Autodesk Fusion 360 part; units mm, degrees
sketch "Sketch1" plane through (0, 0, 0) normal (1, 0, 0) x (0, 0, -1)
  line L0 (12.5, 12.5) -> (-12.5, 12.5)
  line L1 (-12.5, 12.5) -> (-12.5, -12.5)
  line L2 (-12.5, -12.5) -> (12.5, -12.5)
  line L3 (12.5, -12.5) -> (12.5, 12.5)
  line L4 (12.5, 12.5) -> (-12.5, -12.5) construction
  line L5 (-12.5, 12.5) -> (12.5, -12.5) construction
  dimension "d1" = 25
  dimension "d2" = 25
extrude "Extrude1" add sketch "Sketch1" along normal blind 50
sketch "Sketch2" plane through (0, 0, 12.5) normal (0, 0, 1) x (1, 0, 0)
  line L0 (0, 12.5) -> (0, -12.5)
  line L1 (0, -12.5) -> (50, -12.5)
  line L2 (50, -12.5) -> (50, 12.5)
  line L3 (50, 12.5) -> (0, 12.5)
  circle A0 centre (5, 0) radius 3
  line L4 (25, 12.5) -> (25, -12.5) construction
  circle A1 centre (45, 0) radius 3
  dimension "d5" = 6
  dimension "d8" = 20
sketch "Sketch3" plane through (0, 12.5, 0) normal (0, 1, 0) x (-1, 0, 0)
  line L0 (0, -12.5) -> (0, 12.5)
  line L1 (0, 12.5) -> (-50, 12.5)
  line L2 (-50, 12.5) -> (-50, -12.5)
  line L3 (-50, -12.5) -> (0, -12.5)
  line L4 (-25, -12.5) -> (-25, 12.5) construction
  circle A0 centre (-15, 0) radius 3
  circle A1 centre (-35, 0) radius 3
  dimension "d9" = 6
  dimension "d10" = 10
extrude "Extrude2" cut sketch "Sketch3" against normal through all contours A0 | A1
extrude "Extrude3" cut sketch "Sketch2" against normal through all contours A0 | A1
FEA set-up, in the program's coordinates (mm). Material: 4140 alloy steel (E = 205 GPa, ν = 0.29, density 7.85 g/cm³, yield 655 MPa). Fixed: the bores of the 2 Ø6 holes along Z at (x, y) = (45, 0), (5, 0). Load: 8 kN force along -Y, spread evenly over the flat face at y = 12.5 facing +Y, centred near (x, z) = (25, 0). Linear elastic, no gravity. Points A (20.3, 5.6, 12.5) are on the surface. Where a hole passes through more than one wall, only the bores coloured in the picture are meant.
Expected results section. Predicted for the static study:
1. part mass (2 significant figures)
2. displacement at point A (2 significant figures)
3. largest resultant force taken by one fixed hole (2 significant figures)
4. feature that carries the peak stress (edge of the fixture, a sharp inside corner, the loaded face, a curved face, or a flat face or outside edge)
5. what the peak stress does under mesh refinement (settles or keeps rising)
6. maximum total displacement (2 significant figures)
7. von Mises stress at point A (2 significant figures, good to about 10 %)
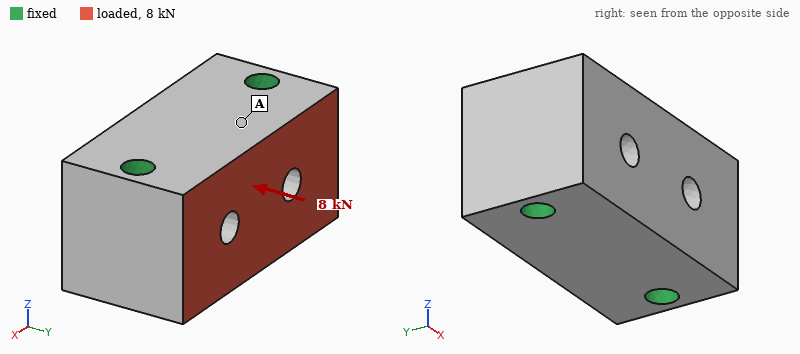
220 g
1.2 µm
4.0 kN
edge of the fixture
keeps rising
1.5 µm
5.5 MPa
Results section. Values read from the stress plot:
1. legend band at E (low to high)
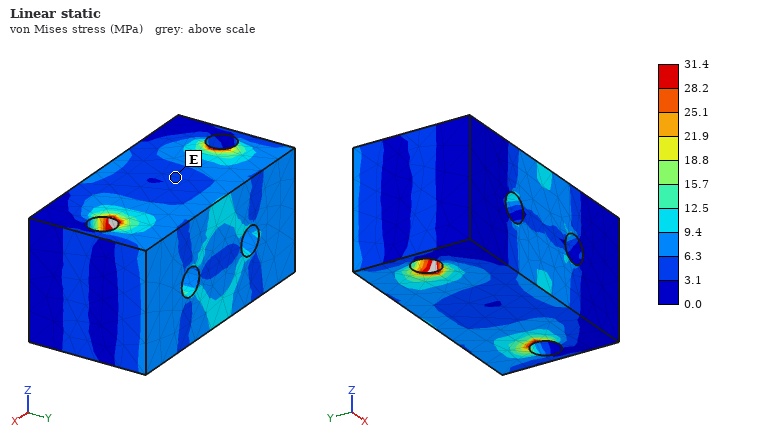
3.1 to 6.3 MPa
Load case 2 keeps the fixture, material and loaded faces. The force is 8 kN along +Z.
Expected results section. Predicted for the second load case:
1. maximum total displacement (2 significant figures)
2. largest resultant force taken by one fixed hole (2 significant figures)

4.4 µm
4.0 kN
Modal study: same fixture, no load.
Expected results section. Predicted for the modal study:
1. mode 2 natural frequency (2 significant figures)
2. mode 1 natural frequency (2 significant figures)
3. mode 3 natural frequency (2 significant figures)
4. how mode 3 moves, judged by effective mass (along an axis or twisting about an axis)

29 kHz
28 kHz
33 kHz
twisting about X
